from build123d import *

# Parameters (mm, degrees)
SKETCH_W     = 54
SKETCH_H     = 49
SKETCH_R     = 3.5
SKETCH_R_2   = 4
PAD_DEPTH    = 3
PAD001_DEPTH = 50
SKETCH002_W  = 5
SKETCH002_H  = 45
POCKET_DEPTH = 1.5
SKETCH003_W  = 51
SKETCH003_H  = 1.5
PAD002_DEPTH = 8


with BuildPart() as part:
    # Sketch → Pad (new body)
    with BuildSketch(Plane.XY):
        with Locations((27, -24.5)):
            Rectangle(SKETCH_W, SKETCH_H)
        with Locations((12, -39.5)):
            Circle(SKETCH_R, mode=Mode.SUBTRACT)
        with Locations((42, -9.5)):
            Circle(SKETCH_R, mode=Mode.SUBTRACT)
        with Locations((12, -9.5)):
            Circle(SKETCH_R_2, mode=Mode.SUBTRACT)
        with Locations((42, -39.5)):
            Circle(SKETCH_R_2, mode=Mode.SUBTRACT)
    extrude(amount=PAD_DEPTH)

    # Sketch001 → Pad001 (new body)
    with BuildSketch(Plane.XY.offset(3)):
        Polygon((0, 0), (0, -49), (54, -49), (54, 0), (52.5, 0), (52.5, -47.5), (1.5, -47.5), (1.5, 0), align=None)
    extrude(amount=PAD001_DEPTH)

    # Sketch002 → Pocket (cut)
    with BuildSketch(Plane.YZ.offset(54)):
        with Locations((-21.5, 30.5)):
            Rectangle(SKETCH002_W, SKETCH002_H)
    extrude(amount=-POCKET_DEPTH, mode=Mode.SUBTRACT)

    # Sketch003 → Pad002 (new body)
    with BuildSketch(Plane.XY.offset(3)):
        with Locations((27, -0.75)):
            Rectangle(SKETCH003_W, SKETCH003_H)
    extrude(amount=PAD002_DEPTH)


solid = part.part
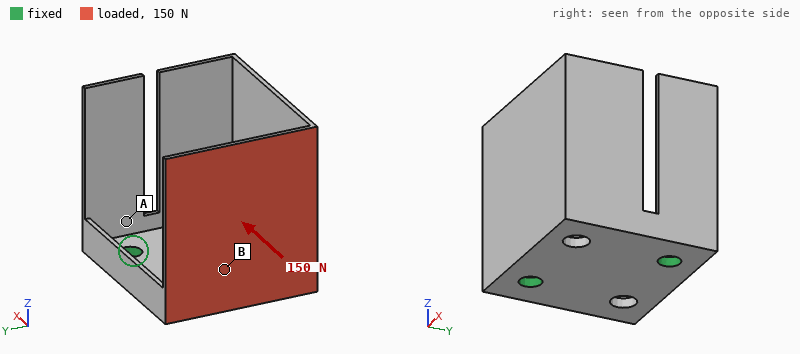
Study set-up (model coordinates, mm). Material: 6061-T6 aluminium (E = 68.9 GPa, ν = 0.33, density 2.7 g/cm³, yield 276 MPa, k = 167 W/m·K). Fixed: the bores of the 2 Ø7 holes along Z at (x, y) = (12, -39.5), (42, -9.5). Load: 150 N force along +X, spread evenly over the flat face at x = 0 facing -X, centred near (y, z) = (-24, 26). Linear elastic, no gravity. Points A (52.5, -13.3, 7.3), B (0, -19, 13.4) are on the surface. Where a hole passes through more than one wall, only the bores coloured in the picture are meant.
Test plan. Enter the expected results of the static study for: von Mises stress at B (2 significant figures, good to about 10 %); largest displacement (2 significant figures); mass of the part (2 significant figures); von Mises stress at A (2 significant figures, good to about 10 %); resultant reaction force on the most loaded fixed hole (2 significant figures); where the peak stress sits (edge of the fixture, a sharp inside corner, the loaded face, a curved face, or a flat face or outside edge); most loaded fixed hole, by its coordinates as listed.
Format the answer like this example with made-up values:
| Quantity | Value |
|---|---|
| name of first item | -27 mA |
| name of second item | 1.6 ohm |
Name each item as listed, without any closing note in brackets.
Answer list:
| Quantity | Value |
|---|---|
| von Mises stress at B | 28 MPa |
| largest displacement | 0.83 mm |
| mass of the part | 51 g |
| von Mises stress at A | 8.7 MPa |
| resultant reaction force on the most loaded fixed hole | 96 N |
| where the peak stress sits | the loaded face |
| most loaded fixed hole, by its coordinates as listed | (12, -39.5) |
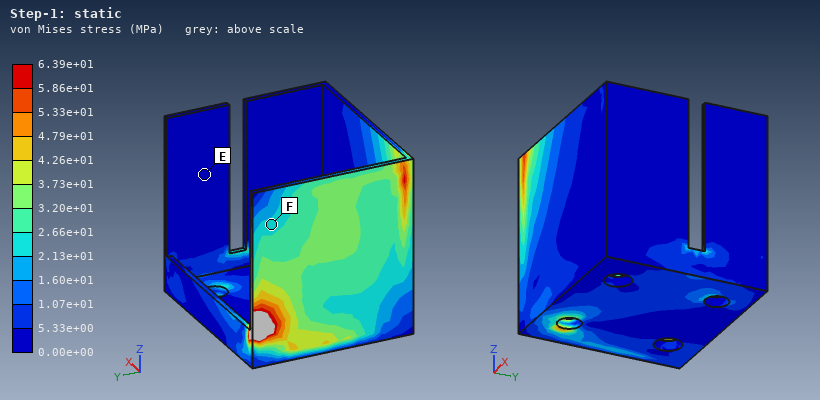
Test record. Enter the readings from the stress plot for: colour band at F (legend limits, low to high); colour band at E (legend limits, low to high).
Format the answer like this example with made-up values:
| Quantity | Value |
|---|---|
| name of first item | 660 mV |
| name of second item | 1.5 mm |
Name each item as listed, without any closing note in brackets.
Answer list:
| Quantity | Value |
|---|---|
| colour band at F | 2.13e+01 to 2.66e+01 MPa |
| colour band at E | 0.00e+00 to 5.33e+00 MPa |
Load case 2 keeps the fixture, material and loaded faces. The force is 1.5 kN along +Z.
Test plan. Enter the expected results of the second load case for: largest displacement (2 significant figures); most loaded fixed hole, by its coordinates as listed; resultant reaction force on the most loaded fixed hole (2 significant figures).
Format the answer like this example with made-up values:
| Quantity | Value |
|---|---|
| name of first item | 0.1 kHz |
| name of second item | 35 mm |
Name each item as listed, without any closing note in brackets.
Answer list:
| Quantity | Value |
|---|---|
| largest displacement | 1.00 mm |
| most loaded fixed hole, by its coordinates as listed | (12, -39.5) |
| resultant reaction force on the most loaded fixed hole | 1.3 kN |
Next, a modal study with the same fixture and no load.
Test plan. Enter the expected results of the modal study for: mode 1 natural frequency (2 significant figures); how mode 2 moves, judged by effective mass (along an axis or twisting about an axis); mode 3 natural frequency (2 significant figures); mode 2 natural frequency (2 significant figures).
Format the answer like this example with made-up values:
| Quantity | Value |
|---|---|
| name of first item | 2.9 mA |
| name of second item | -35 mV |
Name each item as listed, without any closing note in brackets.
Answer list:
| Quantity | Value |
|---|---|
| mode 1 natural frequency | 560 Hz |
| how mode 2 moves, judged by effective mass | along X |
| mode 3 natural frequency | 1200 Hz |
| mode 2 natural frequency | 900 Hz |
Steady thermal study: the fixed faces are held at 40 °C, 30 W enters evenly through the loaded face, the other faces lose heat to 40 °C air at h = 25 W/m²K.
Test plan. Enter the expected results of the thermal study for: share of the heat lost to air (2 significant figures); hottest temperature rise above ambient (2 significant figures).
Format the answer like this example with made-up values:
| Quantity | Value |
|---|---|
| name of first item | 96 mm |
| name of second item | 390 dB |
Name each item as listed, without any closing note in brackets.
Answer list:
| Quantity | Value |
|---|---|
| share of the heat lost to air | 19 % |
| hottest temperature rise above ambient | 52 K |
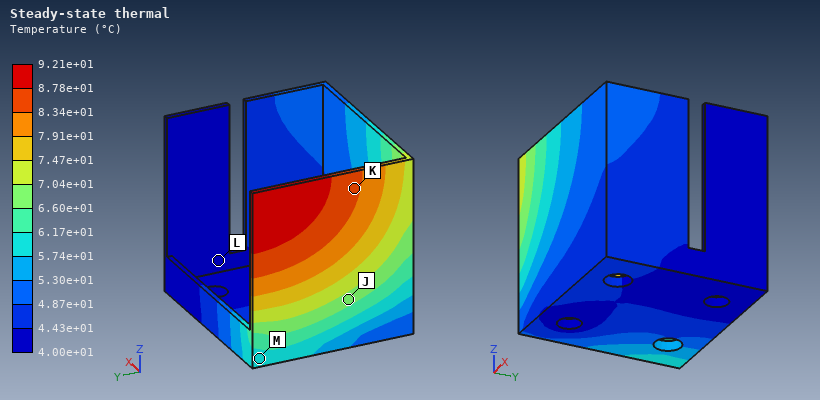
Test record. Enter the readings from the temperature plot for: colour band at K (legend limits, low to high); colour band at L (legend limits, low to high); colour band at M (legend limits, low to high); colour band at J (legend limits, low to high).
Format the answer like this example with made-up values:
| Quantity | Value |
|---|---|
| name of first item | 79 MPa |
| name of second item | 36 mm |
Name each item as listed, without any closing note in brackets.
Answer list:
| Quantity | Value |
|---|---|
| colour band at K | 8.34e+01 to 8.78e+01 °C |
| colour band at L | 4.00e+01 to 4.43e+01 °C |
| colour band at M | 5.74e+01 to 6.17e+01 °C |
| colour band at J | 6.60e+01 to 7.04e+01 °C |
